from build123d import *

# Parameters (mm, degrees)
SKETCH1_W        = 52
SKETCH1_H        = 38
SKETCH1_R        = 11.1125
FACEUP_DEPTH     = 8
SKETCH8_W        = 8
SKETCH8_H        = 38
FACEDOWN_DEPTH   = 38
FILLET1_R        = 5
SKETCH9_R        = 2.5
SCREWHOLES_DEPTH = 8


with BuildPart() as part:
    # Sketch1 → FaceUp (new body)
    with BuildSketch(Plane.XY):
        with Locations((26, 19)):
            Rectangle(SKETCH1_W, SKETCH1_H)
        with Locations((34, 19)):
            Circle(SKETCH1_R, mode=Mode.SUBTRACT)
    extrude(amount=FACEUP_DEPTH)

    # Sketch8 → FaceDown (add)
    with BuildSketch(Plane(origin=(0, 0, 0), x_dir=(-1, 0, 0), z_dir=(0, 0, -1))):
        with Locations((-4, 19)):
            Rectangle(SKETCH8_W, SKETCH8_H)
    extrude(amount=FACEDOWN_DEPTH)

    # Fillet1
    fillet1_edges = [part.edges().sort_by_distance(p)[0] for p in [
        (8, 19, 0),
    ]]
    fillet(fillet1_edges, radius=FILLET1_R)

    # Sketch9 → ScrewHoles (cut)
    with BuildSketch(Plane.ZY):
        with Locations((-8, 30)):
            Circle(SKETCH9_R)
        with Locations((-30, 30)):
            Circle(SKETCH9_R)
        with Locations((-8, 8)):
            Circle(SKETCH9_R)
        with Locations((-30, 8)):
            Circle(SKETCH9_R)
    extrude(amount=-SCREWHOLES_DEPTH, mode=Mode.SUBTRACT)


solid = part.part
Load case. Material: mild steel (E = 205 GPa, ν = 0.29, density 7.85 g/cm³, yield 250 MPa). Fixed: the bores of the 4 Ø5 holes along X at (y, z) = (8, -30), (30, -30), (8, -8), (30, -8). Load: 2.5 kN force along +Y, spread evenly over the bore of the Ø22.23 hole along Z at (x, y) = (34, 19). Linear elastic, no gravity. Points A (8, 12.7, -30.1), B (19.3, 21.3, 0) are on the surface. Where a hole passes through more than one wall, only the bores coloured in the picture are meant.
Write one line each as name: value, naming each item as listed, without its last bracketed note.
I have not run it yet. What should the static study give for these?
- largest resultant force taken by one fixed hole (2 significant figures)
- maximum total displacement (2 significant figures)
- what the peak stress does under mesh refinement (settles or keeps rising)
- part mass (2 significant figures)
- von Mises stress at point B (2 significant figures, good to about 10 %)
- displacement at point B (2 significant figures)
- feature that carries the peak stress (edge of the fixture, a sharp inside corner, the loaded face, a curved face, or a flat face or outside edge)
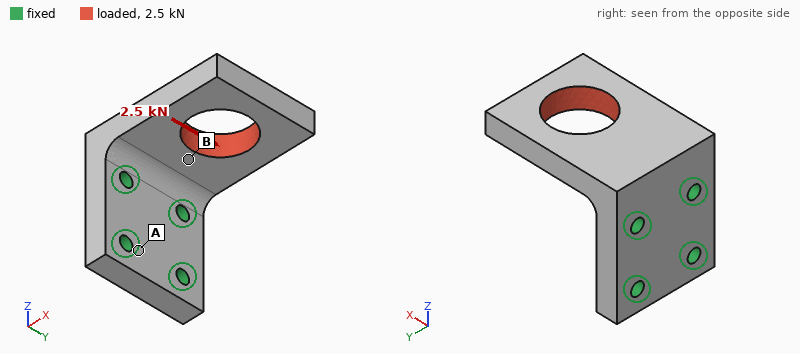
largest resultant force taken by one fixed hole: 3.2 kN
maximum total displacement: 45 µm
what the peak stress does under mesh refinement: keeps rising
part mass: 190 g
von Mises stress at point B: 52 MPa
displacement at point B: 11 µm
feature that carries the peak stress: edge of the fixture
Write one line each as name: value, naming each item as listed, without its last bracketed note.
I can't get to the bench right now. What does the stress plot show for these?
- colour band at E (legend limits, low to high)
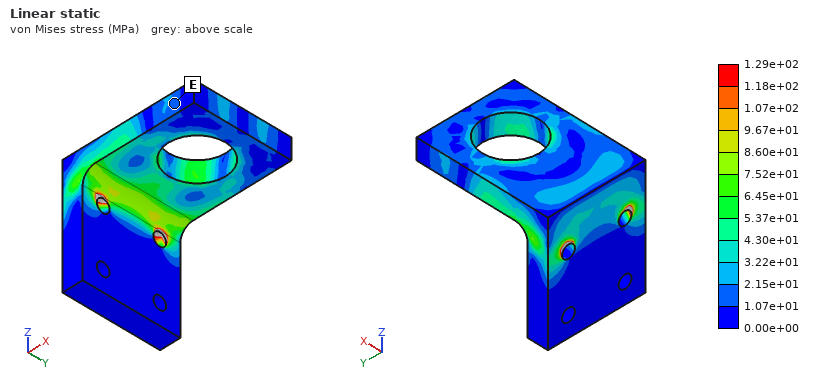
colour band at E: 1.07e+01 to 2.15e+01 MPa
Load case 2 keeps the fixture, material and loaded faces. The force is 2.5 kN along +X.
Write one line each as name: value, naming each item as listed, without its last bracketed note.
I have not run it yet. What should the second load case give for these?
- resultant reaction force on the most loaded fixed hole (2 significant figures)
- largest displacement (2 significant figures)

resultant reaction force on the most loaded fixed hole: 1.4 kN
largest displacement: 27 µm
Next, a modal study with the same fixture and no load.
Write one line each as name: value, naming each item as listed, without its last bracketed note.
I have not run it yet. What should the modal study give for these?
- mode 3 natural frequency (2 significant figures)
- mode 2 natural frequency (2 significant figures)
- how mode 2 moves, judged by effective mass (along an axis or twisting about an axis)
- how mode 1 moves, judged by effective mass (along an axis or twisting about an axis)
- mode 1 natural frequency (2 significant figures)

mode 3 natural frequency: 6800 Hz
mode 2 natural frequency: 5300 Hz
how mode 2 moves, judged by effective mass: along Y
how mode 1 moves, judged by effective mass: along Z
mode 1 natural frequency: 2500 Hz
